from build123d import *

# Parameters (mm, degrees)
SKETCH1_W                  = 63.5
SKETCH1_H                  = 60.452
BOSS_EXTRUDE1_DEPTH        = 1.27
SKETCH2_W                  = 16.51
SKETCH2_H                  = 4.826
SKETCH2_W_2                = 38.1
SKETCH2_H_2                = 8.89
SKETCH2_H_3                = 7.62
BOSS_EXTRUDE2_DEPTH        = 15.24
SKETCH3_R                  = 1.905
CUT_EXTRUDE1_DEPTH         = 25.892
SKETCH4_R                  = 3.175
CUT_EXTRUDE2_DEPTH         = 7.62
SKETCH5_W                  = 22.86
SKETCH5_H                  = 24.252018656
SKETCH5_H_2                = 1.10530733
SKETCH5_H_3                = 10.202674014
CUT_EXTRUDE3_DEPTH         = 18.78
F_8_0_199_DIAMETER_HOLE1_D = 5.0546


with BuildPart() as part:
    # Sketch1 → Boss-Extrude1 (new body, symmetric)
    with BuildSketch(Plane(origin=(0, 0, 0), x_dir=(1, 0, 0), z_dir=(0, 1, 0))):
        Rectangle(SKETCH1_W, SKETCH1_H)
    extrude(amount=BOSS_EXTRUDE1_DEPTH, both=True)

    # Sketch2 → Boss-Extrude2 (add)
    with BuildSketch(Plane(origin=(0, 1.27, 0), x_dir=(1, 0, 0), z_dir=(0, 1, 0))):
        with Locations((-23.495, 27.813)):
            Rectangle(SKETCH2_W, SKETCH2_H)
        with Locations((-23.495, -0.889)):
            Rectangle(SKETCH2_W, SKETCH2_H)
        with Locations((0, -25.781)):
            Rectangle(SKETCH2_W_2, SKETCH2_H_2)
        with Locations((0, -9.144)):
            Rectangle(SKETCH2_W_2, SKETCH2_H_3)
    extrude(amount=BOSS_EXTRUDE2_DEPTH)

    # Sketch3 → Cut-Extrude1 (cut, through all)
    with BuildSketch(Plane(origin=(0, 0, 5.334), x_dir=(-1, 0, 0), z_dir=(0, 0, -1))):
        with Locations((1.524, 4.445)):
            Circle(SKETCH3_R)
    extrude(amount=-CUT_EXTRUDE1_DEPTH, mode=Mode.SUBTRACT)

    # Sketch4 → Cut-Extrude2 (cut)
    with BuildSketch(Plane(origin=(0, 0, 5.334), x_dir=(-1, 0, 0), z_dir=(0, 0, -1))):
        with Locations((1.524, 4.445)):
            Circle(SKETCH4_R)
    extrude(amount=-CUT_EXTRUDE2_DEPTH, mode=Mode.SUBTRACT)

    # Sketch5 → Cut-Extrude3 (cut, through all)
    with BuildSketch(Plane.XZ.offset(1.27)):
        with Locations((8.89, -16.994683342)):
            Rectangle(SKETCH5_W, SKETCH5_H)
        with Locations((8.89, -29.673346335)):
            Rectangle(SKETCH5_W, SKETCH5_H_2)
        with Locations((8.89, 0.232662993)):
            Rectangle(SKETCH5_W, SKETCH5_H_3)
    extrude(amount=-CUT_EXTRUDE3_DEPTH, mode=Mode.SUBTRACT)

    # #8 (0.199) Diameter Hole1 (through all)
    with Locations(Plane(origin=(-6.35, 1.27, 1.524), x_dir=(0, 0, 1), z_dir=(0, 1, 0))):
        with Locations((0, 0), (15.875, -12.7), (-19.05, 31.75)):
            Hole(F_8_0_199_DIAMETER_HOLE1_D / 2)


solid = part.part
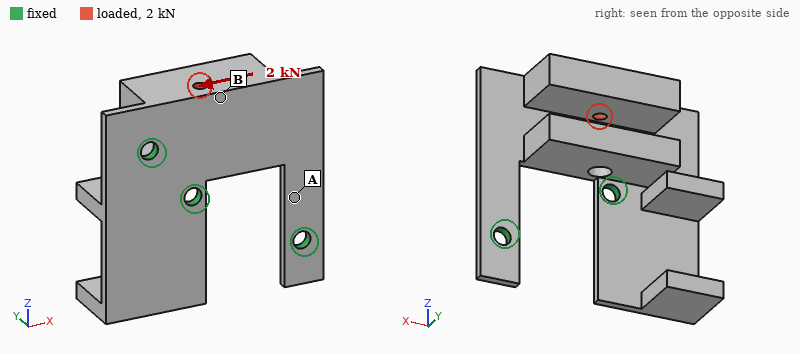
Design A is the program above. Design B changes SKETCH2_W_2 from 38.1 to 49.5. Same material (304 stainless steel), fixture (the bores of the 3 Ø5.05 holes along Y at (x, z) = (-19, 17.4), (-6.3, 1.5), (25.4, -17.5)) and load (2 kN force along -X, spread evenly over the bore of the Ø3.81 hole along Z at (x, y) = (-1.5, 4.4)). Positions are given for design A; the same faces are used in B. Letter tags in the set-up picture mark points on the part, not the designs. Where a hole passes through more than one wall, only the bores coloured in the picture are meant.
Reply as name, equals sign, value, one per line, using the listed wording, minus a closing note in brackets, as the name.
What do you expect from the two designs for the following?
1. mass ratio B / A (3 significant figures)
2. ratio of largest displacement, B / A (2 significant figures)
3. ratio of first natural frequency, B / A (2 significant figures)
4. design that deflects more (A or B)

mass ratio B / A = 1.15
ratio of largest displacement, B / A = 0.67
ratio of first natural frequency, B / A = 1.0
design that deflects more = A
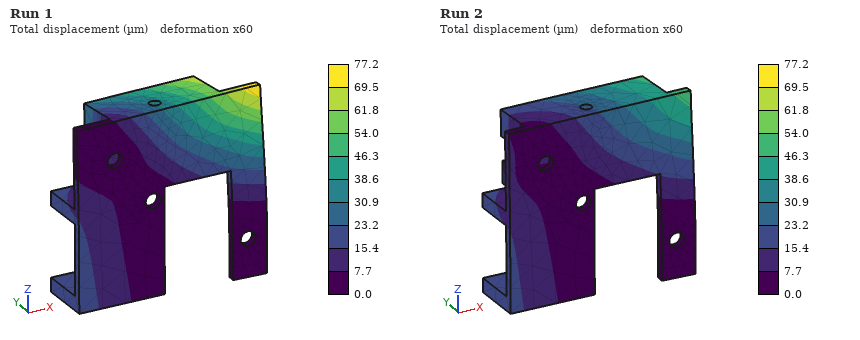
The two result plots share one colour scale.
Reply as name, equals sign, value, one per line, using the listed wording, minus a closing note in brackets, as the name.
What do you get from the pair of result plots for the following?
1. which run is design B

which run is design B = Run 2
